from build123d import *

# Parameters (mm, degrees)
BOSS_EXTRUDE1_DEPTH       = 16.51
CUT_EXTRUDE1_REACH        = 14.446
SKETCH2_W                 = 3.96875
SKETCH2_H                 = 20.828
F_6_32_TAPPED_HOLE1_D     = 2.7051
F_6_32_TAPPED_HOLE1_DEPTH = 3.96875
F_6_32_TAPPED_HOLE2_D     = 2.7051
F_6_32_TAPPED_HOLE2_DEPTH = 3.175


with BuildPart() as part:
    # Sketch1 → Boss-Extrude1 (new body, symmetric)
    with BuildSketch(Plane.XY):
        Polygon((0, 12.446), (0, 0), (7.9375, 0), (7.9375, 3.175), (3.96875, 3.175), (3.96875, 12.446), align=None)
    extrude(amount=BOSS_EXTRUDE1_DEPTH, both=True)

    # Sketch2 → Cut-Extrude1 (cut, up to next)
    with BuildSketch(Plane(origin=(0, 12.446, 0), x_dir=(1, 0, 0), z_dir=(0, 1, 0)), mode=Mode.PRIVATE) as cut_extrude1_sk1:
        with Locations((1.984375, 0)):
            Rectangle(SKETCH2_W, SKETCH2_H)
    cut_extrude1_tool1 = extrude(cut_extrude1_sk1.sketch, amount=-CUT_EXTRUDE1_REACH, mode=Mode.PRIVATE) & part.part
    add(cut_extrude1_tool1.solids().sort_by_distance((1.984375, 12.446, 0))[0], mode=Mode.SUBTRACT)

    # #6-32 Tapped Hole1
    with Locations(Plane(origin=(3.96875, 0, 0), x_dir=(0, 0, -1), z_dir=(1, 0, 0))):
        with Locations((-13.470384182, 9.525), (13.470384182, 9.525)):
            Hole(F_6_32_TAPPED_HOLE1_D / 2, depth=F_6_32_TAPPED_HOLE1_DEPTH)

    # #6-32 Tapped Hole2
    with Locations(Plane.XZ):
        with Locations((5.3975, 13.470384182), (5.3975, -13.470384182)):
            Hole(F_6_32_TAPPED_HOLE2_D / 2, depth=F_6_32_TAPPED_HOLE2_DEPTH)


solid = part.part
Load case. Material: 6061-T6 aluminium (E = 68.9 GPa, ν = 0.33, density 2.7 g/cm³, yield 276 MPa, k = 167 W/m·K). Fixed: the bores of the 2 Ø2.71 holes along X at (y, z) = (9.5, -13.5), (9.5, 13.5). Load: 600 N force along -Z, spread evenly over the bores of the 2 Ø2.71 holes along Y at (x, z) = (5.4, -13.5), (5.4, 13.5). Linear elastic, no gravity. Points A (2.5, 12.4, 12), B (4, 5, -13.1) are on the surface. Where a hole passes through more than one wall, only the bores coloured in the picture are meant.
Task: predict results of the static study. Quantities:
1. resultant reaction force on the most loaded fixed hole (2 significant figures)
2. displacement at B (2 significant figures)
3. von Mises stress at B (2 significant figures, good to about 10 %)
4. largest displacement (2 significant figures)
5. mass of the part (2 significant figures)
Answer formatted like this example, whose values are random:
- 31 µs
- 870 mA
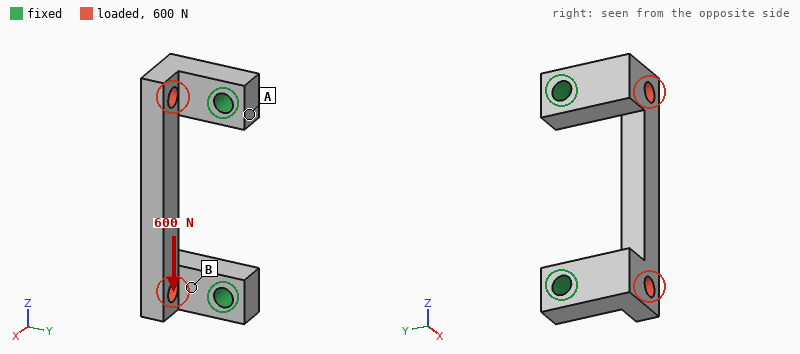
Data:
- 300 N
- 8.4 µm
- 69 MPa
- 27 µm
- 2.5 g
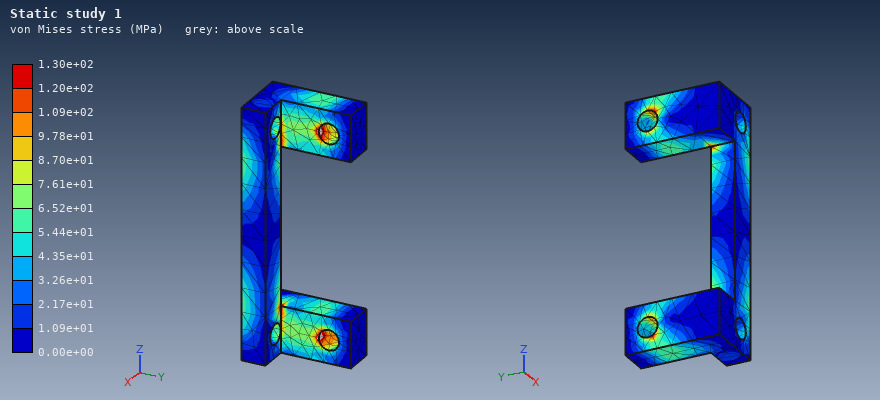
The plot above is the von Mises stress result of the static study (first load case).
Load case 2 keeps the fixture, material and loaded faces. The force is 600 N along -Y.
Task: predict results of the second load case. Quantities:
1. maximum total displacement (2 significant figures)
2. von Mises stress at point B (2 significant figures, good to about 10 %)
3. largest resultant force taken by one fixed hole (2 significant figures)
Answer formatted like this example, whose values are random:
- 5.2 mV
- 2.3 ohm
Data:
- 33 µm
- 80 MPa
- 300 N
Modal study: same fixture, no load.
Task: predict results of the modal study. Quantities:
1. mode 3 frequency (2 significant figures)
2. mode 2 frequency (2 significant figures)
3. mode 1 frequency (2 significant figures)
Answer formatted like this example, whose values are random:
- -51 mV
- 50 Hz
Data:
- 22 kHz
- 22 kHz
- 14 kHz
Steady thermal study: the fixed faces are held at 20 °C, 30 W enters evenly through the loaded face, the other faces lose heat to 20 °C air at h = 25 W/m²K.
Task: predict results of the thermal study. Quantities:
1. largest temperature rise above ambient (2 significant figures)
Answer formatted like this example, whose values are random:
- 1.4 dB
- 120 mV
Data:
- 42 K
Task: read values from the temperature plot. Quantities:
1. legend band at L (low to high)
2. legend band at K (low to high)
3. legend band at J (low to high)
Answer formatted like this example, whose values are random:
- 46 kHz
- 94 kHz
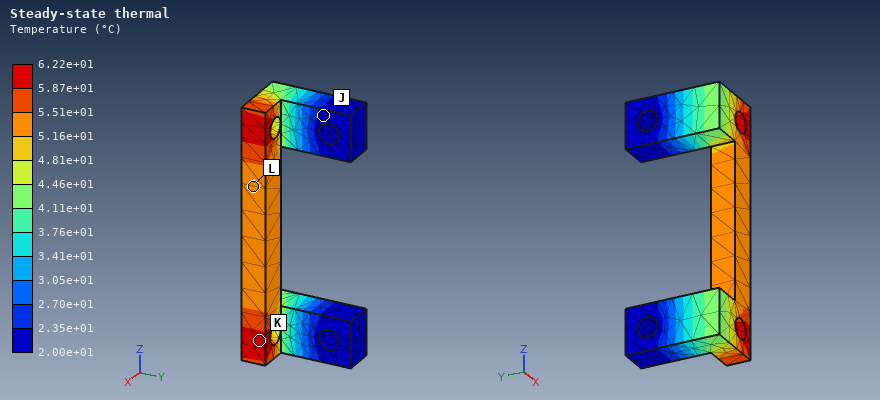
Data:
- 5.16e+01 to 5.51e+01 °C
- 5.87e+01 to 6.22e+01 °C
- 2.00e+01 to 2.35e+01 °C
